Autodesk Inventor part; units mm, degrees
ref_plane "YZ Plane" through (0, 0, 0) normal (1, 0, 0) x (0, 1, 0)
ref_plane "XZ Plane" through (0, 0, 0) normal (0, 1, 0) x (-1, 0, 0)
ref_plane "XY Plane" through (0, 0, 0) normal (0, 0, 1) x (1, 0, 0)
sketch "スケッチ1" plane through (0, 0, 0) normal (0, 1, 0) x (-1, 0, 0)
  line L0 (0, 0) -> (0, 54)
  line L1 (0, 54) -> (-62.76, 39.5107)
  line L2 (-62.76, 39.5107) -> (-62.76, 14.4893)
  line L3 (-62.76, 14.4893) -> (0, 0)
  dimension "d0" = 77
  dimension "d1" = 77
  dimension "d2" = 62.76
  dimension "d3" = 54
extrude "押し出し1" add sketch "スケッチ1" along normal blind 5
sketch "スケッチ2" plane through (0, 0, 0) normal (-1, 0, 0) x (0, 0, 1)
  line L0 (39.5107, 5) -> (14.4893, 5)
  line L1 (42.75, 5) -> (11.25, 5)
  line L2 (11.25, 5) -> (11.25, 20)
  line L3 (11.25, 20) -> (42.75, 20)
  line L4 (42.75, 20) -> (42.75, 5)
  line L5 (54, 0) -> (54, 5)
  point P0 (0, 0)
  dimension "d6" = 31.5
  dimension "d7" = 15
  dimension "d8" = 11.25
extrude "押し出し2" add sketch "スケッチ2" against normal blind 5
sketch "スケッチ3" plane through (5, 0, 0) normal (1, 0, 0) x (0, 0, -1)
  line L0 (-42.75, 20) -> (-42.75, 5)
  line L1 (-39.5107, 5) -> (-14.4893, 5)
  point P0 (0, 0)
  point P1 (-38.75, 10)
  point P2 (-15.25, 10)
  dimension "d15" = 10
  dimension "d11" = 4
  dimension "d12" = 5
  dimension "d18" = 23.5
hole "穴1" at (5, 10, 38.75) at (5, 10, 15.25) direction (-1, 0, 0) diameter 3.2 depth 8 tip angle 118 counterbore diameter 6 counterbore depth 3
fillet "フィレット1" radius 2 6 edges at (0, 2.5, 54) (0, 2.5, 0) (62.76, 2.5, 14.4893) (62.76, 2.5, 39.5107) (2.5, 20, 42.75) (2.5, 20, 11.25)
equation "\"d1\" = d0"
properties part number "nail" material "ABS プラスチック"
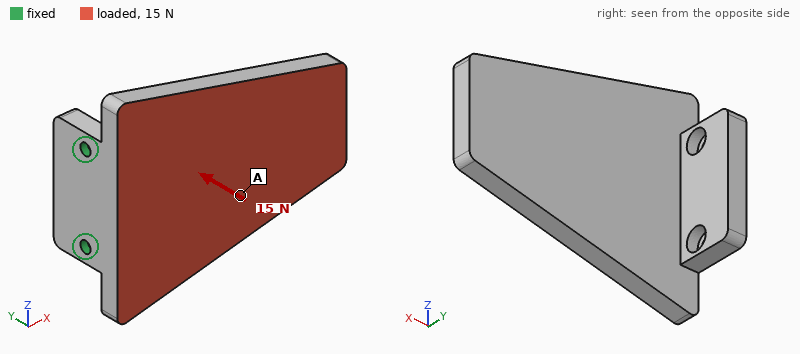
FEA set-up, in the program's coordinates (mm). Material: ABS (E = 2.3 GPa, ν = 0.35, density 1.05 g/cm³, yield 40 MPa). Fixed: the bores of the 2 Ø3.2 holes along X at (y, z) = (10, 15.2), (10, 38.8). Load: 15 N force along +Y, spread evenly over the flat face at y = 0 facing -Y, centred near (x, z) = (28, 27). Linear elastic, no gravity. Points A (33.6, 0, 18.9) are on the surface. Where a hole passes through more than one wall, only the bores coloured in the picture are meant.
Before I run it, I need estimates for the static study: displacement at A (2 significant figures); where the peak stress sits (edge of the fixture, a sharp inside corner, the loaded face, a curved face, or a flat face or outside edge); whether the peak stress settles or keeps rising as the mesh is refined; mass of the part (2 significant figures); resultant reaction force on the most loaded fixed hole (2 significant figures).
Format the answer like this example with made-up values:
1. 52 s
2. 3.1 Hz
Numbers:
1. 0.47 mm
2. edge of the fixture
3. keeps rising
4. 15 g
5. 7.8 N
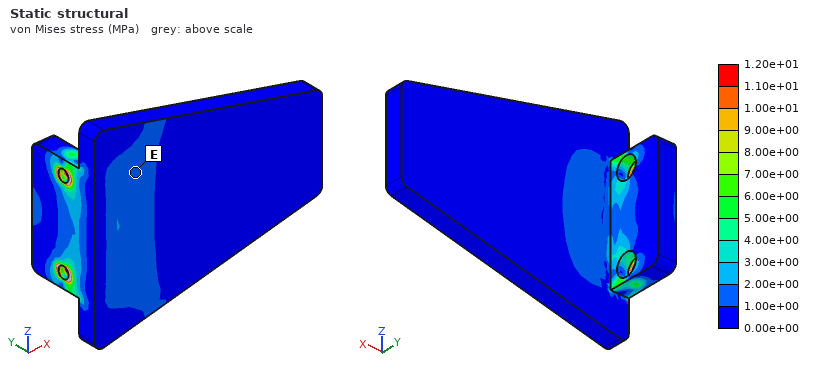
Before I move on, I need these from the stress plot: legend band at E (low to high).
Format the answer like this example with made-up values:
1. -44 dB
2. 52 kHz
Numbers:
1. 1.00e+00 to 2.00e+00 MPa
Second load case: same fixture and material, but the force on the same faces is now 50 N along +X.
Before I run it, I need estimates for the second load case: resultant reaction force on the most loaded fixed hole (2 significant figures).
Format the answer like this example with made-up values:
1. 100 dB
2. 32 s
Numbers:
1. 25 N
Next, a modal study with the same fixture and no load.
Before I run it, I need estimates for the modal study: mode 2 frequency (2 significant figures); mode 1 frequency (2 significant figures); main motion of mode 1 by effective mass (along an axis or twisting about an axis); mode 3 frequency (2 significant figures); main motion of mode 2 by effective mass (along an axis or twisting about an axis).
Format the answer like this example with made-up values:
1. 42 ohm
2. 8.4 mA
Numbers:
1. 780 Hz
2. 220 Hz
3. along Y
4. 1300 Hz
5. along Z
